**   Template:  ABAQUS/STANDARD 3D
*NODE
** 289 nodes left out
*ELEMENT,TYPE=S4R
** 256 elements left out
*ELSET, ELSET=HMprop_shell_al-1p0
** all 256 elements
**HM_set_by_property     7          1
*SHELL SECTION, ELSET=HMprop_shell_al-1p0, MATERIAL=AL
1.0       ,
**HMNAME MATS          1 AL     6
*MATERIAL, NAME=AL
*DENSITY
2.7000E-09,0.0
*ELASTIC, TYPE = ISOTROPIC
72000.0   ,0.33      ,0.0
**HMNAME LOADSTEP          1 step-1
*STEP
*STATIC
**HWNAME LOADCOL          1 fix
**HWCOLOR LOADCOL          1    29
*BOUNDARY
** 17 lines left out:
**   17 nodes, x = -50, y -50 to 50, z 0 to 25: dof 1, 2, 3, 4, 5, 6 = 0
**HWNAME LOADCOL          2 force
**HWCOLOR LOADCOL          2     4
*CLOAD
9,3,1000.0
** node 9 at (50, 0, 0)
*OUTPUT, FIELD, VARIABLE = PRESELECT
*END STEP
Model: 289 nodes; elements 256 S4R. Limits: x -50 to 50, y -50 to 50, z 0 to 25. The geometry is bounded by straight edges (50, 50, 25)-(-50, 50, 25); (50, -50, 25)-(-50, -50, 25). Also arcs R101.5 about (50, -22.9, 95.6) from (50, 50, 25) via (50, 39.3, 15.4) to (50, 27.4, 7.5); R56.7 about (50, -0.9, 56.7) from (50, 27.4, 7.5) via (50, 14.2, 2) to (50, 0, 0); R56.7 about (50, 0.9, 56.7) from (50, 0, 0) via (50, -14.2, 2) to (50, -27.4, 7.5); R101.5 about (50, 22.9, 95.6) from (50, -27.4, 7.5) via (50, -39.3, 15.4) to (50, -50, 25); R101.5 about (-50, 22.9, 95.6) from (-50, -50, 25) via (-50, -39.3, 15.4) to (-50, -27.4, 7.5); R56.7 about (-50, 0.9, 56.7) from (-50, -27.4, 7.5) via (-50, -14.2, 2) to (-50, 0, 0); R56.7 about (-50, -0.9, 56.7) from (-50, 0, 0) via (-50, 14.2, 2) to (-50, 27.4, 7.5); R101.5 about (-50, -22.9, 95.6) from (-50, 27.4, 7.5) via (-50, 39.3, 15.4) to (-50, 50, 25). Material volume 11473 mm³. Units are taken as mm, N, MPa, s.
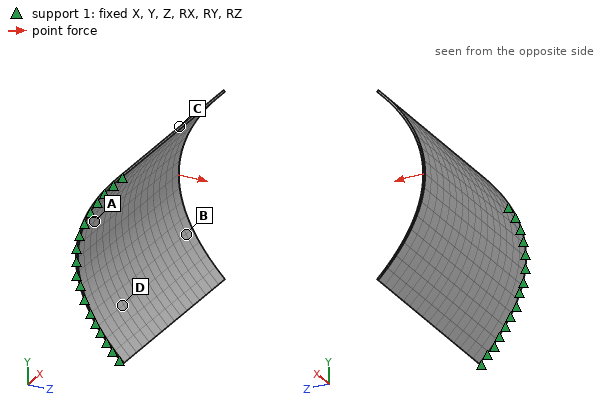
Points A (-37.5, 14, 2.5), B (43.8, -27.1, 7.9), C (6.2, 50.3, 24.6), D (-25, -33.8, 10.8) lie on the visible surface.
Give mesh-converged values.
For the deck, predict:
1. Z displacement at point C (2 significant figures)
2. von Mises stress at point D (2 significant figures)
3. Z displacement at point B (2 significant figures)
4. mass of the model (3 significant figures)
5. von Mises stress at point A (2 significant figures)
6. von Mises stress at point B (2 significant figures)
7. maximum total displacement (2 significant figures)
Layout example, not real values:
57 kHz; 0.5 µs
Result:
-3.1 mm; 150 MPa; -1.9 mm; 0.0310 kg; 140 MPa; 220 MPa; 8.5 mm
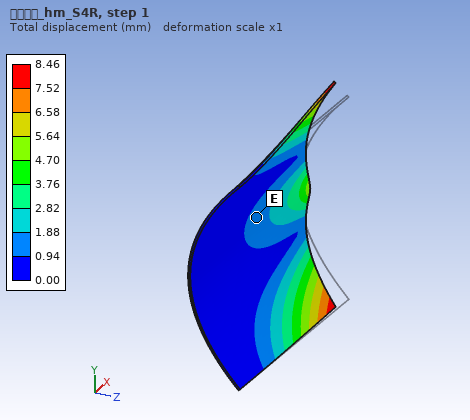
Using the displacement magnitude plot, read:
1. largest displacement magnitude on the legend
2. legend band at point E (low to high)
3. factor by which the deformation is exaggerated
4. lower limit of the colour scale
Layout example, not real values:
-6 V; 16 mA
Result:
8.46 mm; 0.94 to 1.88 mm; 1; 0.00 mm
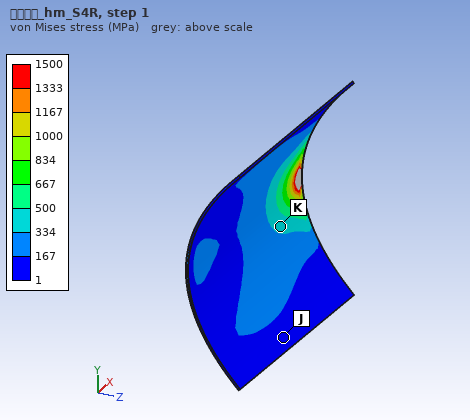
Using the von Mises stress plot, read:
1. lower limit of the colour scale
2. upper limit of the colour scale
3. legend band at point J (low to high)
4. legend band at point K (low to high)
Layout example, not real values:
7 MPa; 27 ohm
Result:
1 MPa; 1500 MPa; 1 to 167 MPa; 334 to 500 MPa
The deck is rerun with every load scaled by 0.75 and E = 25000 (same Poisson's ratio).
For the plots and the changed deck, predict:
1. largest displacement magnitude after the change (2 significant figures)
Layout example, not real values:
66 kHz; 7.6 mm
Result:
18 mm
